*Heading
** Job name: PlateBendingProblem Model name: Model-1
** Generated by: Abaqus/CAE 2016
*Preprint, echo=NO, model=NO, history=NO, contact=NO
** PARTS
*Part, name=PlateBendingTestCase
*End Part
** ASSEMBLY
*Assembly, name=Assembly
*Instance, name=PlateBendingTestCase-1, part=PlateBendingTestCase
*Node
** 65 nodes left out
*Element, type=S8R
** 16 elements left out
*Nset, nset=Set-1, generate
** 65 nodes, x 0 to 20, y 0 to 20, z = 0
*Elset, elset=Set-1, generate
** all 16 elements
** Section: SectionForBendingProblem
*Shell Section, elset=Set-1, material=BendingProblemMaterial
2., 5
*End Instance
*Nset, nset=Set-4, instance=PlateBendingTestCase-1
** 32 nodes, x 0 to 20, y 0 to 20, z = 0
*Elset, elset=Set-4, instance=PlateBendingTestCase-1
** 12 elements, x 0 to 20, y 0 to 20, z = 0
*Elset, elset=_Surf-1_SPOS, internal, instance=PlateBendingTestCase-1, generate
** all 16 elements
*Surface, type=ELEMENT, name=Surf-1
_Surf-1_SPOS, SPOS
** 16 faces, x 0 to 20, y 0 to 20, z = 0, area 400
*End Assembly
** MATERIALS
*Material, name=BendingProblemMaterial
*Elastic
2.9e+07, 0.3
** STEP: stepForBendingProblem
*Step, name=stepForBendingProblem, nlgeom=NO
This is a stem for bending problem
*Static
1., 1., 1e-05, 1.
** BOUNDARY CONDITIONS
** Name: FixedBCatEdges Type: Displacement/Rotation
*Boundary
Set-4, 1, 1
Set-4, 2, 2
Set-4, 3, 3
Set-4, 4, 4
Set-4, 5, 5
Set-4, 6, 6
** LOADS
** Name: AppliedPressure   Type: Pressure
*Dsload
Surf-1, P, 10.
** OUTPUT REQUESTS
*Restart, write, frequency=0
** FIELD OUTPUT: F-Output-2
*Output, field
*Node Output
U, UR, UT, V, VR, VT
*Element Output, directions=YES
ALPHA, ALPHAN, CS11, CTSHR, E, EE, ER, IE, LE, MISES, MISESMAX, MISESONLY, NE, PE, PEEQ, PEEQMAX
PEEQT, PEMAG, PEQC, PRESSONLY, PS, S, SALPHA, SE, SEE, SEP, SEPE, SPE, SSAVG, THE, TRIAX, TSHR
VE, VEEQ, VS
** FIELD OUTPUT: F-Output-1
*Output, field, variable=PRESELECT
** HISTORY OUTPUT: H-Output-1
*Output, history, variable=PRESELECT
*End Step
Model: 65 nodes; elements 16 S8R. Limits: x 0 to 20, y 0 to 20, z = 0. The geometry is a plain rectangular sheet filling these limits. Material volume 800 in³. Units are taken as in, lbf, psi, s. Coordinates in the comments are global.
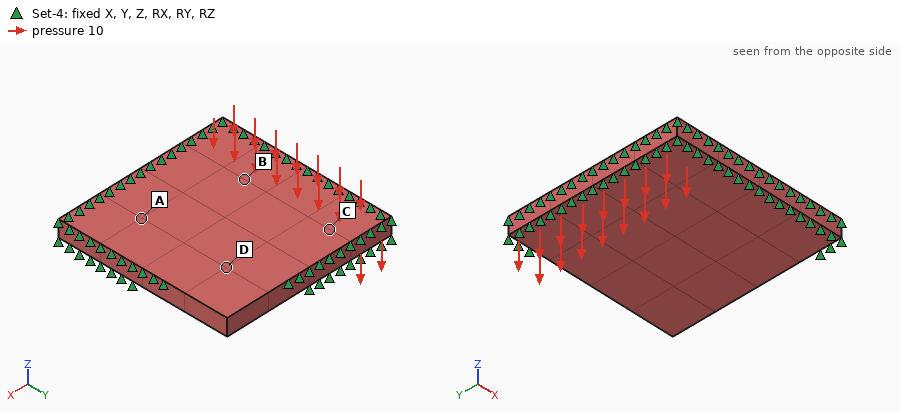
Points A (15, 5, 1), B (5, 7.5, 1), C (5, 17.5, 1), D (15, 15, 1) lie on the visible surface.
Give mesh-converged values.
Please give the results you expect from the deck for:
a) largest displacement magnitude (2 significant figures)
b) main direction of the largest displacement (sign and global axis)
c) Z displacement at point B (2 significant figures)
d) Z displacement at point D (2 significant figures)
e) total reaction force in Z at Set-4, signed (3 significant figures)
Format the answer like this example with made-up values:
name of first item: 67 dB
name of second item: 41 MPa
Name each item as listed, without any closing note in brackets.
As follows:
largest displacement magnitude: 1.0e-04 in
main direction of the largest displacement: -Z
Z displacement at point B: -5.8e-05 in
Z displacement at point D: -4.0e-05 in
total reaction force in Z at Set-4, signed: 4000 lbf
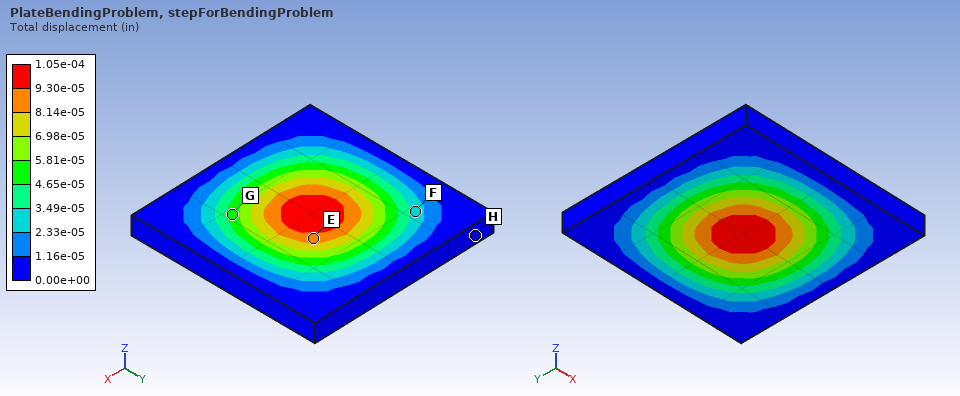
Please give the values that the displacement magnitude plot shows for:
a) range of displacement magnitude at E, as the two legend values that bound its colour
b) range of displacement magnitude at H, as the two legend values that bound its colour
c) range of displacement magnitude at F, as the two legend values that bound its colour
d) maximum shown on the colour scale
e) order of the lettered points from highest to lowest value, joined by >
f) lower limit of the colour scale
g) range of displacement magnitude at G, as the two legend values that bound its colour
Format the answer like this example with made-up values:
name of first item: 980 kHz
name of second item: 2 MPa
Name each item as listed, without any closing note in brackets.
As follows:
range of displacement magnitude at E, as the two legend values that bound its colour: 8.14e-05 to 9.30e-05 in
range of displacement magnitude at H, as the two legend values that bound its colour: 0.00e+00 to 1.16e-05 in
range of displacement magnitude at F, as the two legend values that bound its colour: 2.33e-05 to 3.49e-05 in
maximum shown on the colour scale: 1.05e-04 in
order of the lettered points from highest to lowest value, joined by >: E > G > F > H
lower limit of the colour scale: 0.00e+00 in
range of displacement magnitude at G, as the two legend values that bound its colour: 4.65e-05 to 5.81e-05 in
